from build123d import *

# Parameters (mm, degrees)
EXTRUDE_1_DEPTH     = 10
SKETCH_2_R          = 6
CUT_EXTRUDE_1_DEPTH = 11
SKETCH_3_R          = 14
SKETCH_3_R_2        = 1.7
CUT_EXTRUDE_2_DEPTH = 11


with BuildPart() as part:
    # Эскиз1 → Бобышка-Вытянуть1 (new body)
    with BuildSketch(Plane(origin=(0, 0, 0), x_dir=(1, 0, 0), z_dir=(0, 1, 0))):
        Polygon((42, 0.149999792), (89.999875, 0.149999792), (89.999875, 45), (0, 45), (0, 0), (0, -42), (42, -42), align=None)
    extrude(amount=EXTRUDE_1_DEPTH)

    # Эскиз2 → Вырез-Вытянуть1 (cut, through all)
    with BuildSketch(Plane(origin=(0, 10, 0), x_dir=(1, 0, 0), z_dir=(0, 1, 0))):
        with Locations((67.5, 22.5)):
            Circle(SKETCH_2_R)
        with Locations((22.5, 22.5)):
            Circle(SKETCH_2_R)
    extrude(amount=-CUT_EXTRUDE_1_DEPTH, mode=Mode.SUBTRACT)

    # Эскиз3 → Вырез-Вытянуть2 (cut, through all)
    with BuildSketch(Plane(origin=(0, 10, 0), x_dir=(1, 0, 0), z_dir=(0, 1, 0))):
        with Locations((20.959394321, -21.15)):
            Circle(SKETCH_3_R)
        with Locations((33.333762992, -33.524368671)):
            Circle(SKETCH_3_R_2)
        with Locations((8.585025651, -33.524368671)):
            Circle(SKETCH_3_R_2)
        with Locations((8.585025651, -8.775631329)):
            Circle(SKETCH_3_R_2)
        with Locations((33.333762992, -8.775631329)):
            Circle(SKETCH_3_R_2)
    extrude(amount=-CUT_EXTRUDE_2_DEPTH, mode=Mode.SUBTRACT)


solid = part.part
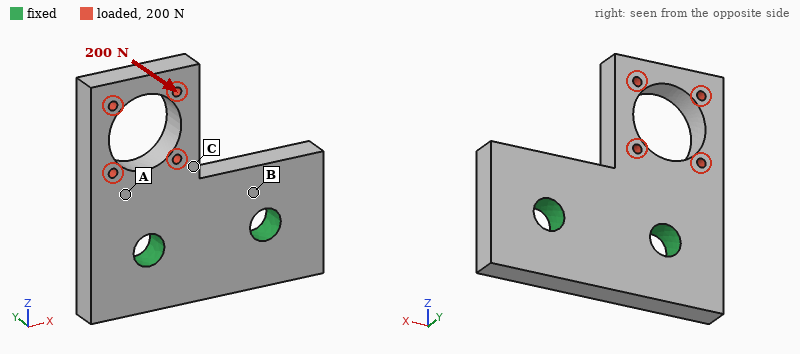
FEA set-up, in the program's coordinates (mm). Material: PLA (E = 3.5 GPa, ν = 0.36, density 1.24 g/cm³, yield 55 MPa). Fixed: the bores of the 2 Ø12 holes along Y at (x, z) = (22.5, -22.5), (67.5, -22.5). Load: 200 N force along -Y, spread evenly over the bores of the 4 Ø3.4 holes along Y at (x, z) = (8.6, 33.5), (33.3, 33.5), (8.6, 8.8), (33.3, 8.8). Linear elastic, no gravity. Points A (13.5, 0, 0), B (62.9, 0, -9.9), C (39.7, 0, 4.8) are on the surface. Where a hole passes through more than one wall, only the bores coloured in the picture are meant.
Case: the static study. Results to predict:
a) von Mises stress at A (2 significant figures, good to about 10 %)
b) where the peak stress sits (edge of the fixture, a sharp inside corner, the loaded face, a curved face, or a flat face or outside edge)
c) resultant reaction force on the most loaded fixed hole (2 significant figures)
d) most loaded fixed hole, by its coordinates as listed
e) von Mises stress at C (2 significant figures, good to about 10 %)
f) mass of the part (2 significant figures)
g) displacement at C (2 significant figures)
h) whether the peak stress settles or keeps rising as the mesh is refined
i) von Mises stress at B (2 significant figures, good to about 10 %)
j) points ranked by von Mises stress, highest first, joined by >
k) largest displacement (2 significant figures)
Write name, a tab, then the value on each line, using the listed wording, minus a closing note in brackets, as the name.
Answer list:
von Mises stress at A	5.1 MPa
where the peak stress sits	edge of the fixture
resultant reaction force on the most loaded fixed hole	200 N
most loaded fixed hole, by its coordinates as listed	(22.5, -22.5)
von Mises stress at C	8.9 MPa
mass of the part	61 g
displacement at C	0.14 mm
whether the peak stress settles or keeps rising as the mesh is refined	keeps rising
von Mises stress at B	2.0 MPa
points ranked by von Mises stress, highest first, joined by >	C > A > B
largest displacement	0.84 mm
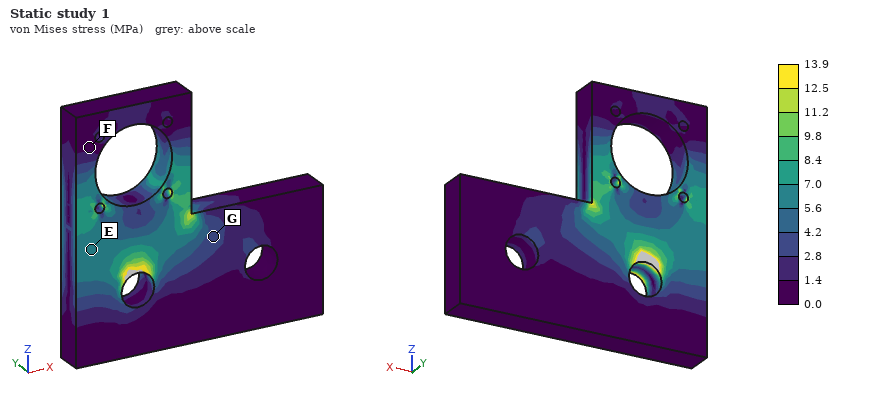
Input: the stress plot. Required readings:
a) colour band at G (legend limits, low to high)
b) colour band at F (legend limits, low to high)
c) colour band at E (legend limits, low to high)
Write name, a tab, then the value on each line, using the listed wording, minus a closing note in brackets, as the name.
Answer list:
colour band at G	2.8 to 4.2 MPa
colour band at F	0.0 to 1.4 MPa
colour band at E	5.6 to 7.0 MPa
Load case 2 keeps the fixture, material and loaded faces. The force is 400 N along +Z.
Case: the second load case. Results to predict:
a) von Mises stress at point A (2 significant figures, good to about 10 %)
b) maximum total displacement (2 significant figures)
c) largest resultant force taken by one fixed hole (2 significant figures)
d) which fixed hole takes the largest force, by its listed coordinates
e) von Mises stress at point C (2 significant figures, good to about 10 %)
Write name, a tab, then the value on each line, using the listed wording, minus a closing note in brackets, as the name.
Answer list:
von Mises stress at point A	1.1 MPa
maximum total displacement	42 µm
largest resultant force taken by one fixed hole	380 N
which fixed hole takes the largest force, by its listed coordinates	(22.5, -22.5)
von Mises stress at point C	1.9 MPa
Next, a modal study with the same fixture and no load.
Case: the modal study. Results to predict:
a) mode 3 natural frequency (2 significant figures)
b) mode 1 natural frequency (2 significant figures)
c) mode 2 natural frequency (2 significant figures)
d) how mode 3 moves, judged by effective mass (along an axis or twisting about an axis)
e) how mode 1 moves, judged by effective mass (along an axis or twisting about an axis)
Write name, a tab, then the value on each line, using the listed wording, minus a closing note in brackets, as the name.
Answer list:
mode 3 natural frequency	1900 Hz
mode 1 natural frequency	790 Hz
mode 2 natural frequency	1700 Hz
how mode 3 moves, judged by effective mass	along X
how mode 1 moves, judged by effective mass	along Y
